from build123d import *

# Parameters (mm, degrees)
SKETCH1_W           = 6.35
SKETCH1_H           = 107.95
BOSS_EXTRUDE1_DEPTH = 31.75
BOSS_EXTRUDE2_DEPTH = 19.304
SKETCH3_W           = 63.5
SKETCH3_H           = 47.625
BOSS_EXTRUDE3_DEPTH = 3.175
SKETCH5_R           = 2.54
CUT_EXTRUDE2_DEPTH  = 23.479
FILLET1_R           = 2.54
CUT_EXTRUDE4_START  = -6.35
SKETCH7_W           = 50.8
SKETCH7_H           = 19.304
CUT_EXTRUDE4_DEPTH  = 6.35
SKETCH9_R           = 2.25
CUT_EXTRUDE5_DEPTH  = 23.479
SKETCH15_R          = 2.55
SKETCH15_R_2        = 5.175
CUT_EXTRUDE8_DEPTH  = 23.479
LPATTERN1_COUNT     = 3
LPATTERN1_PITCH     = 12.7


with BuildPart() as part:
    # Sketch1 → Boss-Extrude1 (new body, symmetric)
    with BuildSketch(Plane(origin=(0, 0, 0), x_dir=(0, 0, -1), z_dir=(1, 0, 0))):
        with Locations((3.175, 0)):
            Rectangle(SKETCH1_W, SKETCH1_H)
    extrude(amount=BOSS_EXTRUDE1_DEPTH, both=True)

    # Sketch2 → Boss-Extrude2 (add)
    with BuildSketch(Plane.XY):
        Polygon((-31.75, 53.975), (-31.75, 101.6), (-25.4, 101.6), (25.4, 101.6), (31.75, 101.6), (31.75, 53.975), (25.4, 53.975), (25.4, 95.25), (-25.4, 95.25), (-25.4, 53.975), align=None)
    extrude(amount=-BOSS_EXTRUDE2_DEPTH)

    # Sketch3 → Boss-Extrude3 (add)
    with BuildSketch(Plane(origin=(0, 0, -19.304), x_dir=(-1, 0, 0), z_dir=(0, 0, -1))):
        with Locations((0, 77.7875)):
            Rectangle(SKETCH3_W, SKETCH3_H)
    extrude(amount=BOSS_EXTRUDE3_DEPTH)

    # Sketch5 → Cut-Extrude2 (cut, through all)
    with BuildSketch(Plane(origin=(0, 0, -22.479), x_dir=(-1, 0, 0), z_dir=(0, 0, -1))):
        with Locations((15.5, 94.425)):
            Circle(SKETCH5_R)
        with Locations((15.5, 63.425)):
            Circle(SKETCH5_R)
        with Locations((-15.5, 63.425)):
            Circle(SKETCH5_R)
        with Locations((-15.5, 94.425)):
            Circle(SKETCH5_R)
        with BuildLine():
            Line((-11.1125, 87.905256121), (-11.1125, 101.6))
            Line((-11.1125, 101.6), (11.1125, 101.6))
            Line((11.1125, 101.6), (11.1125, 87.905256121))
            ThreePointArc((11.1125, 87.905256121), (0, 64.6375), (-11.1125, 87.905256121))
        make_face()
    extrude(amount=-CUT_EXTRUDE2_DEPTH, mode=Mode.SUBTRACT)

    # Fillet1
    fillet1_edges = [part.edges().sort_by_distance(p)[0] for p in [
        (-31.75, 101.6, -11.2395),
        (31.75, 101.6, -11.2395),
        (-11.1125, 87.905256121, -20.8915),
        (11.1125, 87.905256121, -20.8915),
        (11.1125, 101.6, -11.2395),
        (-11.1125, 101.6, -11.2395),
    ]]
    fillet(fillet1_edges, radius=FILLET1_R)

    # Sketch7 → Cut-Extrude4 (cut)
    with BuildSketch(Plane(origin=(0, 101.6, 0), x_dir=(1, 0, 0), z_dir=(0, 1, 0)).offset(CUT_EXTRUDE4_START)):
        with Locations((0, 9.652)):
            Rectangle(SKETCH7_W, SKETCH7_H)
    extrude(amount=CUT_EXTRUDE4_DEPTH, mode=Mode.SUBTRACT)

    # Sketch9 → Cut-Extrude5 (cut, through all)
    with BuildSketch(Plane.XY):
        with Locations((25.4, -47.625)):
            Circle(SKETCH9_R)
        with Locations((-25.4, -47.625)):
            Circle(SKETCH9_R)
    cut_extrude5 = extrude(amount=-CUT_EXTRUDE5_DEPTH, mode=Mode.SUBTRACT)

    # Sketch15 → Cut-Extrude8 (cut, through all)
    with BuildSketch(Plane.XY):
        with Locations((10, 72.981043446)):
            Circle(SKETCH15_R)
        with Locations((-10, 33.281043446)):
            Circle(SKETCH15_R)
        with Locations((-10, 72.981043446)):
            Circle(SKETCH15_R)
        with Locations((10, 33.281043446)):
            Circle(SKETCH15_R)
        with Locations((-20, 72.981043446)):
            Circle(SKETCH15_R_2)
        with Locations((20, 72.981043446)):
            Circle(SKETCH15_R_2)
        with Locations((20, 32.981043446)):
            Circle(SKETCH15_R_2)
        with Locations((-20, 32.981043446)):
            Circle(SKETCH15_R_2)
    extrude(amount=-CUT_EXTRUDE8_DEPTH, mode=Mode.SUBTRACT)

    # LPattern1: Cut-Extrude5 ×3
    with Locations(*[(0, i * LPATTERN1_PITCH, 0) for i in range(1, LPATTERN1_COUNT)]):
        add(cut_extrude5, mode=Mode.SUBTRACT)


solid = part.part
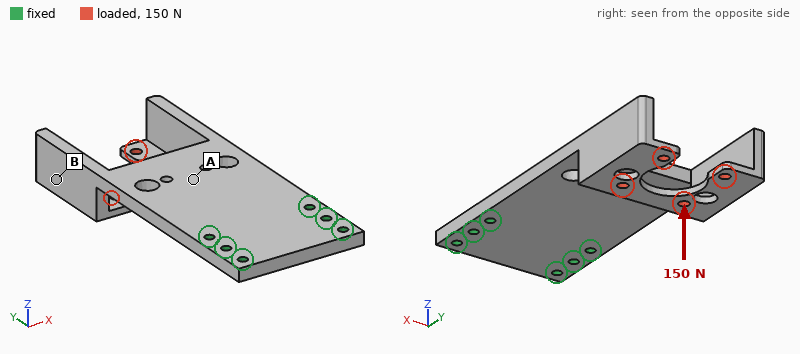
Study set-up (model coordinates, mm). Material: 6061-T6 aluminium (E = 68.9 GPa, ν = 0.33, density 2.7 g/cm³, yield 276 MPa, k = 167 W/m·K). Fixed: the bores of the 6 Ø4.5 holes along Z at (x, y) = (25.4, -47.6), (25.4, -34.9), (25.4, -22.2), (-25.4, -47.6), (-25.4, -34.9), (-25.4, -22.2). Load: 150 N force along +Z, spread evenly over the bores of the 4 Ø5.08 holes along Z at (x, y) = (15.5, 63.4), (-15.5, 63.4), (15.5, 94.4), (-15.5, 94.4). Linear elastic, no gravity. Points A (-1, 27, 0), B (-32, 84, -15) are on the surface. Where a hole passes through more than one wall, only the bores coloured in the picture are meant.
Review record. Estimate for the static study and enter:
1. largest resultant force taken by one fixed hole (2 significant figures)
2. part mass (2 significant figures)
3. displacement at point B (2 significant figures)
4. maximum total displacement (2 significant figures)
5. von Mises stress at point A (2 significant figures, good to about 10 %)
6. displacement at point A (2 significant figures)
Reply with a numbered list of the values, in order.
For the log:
1. 280 N
2. 160 g
3. 0.73 mm
4. 0.94 mm
5. 22 MPa
6. 0.19 mm
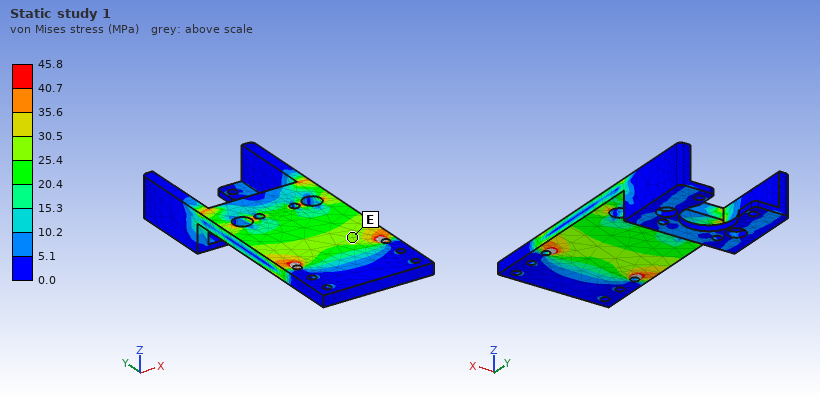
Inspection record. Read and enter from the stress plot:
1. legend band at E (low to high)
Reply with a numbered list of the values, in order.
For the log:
1. 25.4 to 30.5 MPa
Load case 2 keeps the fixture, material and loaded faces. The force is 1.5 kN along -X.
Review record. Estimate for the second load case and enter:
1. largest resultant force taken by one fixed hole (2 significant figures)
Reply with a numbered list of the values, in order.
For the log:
1. 2.6 kN
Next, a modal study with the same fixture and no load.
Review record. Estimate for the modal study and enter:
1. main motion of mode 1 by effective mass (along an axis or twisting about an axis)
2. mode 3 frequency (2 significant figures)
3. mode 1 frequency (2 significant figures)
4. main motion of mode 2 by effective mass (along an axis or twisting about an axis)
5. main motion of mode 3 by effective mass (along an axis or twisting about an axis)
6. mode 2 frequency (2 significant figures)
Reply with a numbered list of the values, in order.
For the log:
1. along Z
2. 1400 Hz
3. 320 Hz
4. twisting about Y
5. along X
6. 760 Hz
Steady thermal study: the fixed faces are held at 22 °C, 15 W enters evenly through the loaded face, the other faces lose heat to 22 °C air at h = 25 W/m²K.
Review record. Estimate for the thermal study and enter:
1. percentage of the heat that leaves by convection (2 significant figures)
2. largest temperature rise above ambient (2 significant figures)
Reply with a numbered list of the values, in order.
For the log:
1. 45 %
2. 29 K
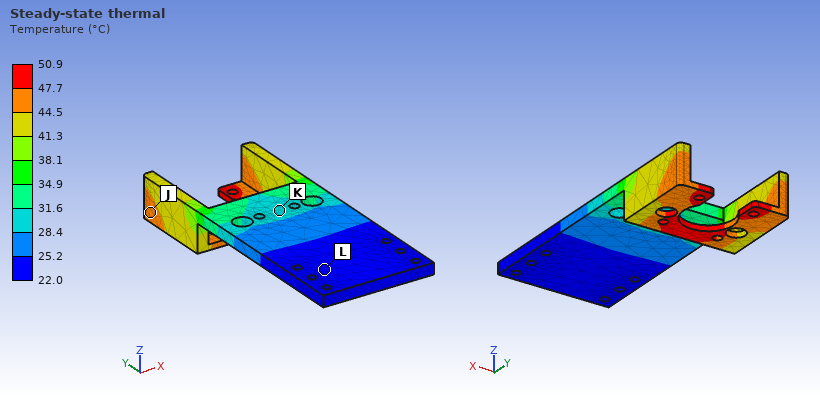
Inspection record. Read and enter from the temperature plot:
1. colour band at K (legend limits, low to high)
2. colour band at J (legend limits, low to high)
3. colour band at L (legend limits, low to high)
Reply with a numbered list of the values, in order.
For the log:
1. 28.4 to 31.6 °C
2. 44.5 to 47.7 °C
3. 22.0 to 25.2 °C
